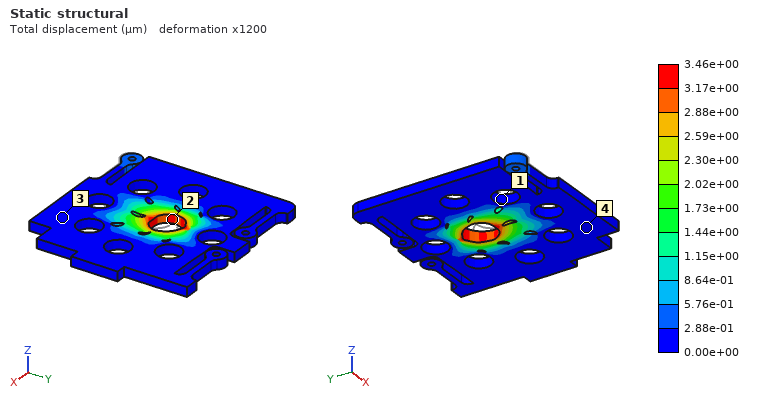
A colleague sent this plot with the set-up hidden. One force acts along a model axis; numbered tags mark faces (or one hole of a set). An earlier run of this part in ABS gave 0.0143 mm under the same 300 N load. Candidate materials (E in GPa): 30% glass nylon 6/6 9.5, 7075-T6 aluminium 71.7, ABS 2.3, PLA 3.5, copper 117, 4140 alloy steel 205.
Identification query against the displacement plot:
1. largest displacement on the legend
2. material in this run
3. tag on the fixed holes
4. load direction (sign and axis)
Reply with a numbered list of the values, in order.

1. 3.46e+00 µm
2. 30% glass nylon 6/6
3. 1
4. +Y
